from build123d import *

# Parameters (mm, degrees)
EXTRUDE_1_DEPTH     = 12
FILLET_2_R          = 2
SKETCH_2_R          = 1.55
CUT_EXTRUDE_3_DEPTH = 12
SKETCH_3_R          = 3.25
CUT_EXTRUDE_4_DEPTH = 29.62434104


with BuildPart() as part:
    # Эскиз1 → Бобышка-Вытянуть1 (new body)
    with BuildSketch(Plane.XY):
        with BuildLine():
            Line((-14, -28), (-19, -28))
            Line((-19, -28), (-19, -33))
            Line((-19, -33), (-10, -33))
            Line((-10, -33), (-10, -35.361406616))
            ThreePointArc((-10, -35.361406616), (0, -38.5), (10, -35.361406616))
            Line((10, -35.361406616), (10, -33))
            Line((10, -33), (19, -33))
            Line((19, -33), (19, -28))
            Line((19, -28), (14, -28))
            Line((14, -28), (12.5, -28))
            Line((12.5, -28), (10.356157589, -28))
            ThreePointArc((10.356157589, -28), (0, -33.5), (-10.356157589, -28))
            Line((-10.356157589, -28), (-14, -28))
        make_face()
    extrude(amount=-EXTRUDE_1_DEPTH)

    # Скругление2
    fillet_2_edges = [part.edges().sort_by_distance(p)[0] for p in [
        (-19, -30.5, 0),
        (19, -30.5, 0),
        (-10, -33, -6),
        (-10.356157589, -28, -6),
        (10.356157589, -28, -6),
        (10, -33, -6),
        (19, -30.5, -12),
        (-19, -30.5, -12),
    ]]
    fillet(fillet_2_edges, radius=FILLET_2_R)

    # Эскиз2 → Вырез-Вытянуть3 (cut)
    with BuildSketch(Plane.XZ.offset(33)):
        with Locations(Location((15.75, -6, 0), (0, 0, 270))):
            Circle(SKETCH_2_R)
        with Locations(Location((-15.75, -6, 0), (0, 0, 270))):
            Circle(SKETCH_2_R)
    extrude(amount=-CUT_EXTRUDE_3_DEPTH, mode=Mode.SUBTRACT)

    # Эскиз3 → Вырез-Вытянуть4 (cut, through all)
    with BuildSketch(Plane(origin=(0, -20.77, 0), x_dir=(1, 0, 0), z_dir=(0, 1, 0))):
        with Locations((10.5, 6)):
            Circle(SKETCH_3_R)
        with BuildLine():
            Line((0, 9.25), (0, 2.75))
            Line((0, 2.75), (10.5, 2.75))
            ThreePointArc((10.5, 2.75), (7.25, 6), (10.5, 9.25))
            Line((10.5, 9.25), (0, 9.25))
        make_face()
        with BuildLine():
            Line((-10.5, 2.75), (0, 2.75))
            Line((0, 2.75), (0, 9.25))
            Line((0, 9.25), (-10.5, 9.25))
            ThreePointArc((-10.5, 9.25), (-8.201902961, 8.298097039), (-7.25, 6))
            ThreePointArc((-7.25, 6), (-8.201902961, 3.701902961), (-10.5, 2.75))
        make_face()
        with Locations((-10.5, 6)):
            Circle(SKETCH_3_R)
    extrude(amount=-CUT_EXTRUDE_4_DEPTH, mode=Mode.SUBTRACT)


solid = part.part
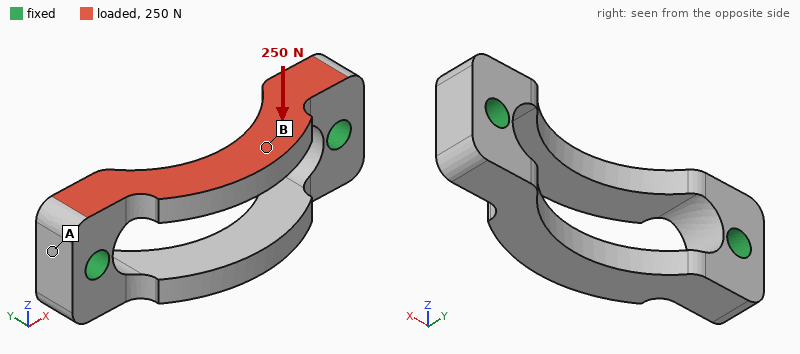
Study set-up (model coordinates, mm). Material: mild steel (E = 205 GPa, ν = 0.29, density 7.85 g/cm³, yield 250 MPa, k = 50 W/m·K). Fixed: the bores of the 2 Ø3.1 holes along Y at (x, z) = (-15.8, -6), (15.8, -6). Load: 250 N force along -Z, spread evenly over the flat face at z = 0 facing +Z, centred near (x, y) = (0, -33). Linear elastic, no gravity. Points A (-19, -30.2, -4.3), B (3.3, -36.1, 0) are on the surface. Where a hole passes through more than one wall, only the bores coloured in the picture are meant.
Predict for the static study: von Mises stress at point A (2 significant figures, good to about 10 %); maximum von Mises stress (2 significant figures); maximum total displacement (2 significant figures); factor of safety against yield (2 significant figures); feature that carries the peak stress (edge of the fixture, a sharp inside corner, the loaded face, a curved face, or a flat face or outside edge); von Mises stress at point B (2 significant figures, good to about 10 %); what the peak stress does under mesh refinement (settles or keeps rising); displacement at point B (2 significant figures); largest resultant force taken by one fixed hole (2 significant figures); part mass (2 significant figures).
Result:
12 MPa
140 MPa
15 µm
1.8
a curved face
32 MPa
settles
11 µm
130 N
11 g
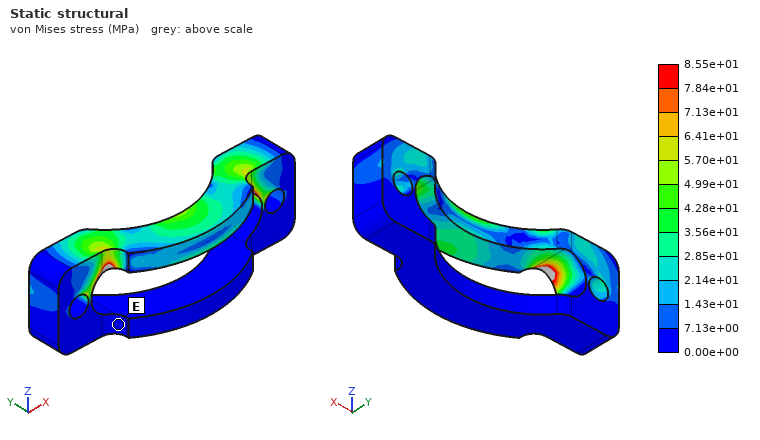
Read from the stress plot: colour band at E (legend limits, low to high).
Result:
0.00e+00 to 7.13e+00 MPa
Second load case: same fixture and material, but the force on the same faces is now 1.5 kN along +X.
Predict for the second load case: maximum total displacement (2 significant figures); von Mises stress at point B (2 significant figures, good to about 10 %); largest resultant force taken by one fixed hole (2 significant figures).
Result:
6.4 µm
44 MPa
760 N
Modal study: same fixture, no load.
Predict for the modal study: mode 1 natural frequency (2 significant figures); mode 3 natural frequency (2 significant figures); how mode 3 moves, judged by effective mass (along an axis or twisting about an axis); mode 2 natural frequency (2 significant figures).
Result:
13 kHz
29 kHz
twisting about X
13 kHz
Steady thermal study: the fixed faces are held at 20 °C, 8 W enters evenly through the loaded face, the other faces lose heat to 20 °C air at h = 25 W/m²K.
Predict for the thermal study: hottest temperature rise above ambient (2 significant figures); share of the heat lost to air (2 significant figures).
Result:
47 K
3.6 %
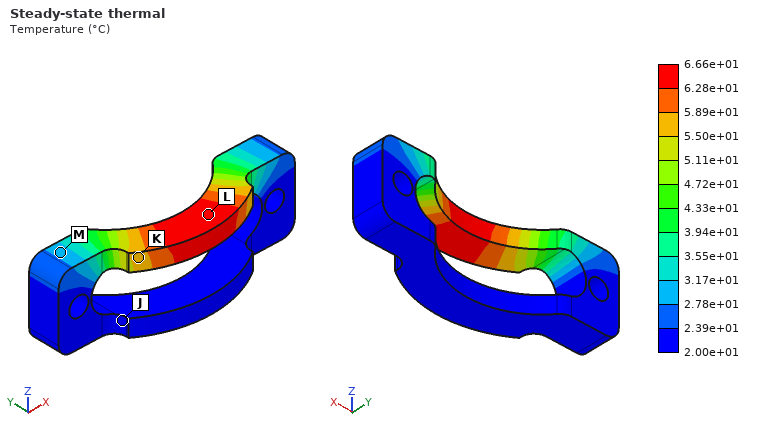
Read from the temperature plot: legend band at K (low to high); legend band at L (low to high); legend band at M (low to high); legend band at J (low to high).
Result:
5.50e+01 to 5.89e+01 °C
6.28e+01 to 6.66e+01 °C
2.78e+01 to 3.17e+01 °C
2.00e+01 to 2.39e+01 °C
